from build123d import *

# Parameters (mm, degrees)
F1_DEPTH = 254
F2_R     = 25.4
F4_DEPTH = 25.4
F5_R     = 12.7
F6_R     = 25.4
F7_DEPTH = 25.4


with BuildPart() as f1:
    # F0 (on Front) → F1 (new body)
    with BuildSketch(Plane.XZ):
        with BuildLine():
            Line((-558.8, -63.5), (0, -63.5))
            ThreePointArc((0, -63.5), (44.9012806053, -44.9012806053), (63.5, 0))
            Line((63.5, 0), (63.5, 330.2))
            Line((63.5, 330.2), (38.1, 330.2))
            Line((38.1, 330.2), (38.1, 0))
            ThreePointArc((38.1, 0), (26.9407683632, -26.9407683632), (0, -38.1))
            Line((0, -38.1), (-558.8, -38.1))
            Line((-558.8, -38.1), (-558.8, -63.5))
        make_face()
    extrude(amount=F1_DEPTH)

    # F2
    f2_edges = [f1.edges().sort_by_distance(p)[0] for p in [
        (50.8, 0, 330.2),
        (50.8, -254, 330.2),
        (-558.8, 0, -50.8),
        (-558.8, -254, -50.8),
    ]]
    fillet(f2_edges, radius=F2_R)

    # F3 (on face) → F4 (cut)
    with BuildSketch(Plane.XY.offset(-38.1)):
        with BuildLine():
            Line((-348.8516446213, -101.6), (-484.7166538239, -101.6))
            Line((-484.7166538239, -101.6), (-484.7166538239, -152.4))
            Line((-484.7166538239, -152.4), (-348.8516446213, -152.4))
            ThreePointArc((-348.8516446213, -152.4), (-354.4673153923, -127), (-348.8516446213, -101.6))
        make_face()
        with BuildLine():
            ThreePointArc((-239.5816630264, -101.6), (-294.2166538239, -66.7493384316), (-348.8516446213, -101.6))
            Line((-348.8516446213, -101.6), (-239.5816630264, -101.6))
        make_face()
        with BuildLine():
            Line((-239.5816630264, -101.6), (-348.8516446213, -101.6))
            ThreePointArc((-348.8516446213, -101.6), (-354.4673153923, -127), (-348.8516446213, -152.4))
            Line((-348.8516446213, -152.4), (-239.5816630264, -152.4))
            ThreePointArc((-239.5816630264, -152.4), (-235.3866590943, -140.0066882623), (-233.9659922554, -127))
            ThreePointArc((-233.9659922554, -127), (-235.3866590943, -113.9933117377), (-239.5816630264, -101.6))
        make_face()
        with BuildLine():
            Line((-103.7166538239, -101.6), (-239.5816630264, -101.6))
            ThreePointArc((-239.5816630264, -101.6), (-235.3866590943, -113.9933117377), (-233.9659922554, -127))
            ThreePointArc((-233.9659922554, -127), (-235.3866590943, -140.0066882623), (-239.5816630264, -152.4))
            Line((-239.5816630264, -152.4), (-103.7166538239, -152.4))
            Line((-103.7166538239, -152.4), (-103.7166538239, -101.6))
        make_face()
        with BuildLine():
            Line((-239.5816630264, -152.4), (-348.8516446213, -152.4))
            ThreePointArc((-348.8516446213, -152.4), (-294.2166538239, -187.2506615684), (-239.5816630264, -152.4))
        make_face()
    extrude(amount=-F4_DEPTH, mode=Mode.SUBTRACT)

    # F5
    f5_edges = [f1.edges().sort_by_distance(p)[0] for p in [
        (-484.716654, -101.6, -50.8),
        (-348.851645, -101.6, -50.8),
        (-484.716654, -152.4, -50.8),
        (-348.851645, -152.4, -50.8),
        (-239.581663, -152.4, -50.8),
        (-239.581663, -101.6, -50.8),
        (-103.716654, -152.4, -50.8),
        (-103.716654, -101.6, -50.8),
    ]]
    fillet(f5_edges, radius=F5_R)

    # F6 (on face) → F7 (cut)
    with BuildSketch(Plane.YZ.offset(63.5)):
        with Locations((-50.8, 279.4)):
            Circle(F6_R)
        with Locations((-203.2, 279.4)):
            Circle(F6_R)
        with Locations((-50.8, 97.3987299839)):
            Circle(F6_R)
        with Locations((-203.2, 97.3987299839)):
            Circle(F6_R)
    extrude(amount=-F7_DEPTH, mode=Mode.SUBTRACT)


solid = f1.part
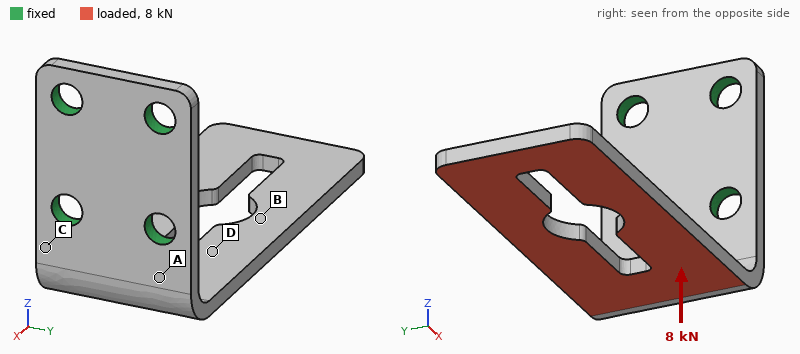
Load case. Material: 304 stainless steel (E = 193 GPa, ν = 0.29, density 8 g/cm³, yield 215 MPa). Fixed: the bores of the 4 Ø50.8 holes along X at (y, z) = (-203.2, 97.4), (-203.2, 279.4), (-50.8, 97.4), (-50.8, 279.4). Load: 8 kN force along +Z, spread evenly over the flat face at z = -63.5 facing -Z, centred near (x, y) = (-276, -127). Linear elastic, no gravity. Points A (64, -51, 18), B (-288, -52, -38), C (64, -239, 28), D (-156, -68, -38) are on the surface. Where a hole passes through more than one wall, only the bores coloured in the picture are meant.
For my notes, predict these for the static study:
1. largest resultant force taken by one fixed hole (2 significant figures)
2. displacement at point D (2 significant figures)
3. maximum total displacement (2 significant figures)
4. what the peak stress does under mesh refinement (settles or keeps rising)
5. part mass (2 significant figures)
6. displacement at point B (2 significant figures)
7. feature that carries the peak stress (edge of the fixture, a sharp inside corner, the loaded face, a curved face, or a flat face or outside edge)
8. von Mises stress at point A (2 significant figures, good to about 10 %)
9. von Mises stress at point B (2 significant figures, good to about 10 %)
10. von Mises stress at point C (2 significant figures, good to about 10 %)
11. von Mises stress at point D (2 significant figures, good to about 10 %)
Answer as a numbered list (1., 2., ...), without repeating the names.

1. 4.7 kN
2. 1.5 mm
3. 6.5 mm
4. keeps rising
5. 43 kg
6. 2.9 mm
7. edge of the fixture
8. 83 MPa
9. 40 MPa
10. 97 MPa
11. 53 MPa
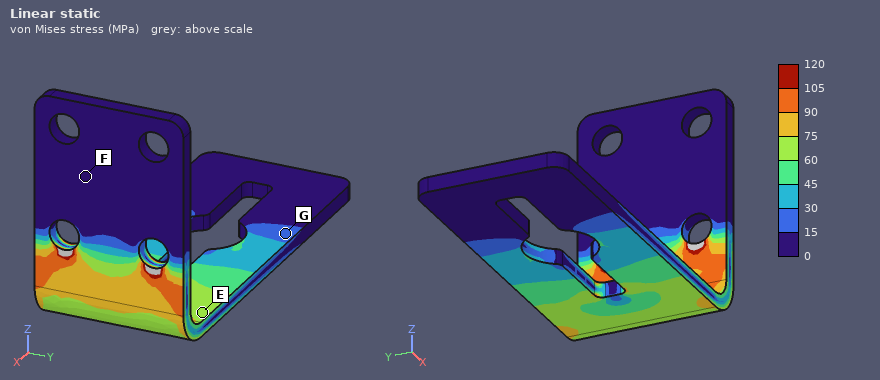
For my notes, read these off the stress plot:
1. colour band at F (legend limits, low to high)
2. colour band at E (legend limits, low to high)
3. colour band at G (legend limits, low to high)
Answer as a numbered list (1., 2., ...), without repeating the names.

1. 0 to 15 MPa
2. 60 to 75 MPa
3. 15 to 30 MPa
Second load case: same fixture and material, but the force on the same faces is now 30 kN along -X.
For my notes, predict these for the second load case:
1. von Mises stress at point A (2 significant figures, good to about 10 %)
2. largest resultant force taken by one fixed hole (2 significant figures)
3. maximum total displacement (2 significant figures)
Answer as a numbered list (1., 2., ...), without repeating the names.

1. 80 MPa
2. 15 kN
3. 3.6 mm
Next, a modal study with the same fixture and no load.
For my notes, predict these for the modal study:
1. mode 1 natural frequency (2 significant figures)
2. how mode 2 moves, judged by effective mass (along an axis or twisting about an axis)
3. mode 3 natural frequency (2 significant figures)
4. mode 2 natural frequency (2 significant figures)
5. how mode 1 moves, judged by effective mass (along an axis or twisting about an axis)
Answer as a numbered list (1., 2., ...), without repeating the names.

1. 44 Hz
2. along Y
3. 230 Hz
4. 110 Hz
5. along Z
